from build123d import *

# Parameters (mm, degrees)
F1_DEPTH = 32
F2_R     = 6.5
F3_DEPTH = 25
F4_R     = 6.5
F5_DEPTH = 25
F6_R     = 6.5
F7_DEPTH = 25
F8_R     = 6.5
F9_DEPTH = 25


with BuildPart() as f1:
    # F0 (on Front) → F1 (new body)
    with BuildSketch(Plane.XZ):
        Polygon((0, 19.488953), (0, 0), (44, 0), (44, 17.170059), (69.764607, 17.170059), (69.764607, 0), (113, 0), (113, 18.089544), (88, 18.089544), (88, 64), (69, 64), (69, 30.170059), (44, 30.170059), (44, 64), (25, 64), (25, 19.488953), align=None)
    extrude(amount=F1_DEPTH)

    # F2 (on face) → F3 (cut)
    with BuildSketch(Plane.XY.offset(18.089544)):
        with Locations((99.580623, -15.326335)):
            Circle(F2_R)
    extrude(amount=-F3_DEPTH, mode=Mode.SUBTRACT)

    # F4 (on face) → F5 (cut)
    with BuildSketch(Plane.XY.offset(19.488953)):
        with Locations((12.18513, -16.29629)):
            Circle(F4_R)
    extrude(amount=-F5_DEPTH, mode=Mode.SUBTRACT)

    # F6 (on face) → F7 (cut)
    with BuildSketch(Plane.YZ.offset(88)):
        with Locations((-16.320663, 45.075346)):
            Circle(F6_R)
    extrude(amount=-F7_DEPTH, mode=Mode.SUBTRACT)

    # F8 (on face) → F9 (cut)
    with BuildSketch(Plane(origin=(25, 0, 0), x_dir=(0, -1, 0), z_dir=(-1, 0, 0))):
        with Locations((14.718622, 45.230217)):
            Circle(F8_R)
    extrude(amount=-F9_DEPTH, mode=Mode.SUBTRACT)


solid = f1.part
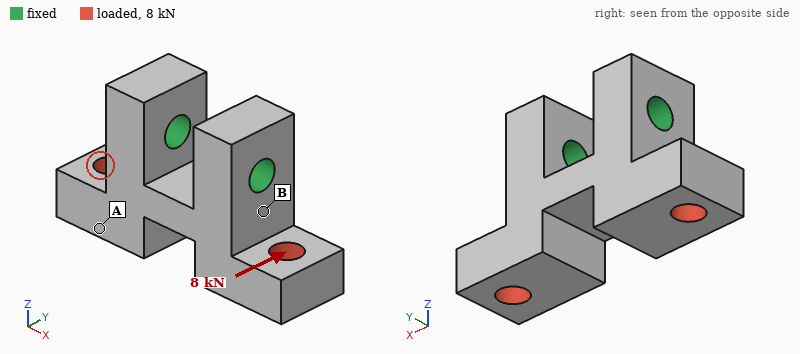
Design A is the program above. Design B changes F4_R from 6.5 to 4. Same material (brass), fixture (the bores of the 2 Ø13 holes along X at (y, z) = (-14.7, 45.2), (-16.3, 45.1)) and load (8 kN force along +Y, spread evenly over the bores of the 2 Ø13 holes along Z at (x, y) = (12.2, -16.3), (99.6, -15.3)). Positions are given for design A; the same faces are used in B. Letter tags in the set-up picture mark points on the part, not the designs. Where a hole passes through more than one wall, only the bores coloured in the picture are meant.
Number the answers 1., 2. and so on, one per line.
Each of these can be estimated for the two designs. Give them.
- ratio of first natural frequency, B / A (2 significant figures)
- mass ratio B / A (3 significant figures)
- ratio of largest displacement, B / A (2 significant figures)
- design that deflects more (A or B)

1. 0.97
2. 1.01
3. 1.2
4. B
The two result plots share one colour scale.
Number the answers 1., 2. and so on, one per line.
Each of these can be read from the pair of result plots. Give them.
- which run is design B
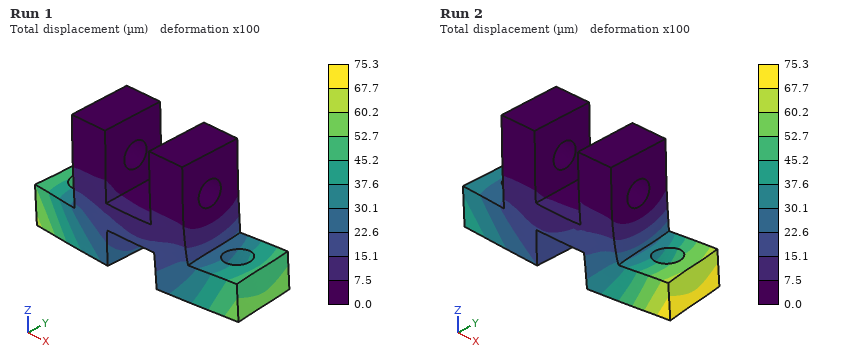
1. Run 2
